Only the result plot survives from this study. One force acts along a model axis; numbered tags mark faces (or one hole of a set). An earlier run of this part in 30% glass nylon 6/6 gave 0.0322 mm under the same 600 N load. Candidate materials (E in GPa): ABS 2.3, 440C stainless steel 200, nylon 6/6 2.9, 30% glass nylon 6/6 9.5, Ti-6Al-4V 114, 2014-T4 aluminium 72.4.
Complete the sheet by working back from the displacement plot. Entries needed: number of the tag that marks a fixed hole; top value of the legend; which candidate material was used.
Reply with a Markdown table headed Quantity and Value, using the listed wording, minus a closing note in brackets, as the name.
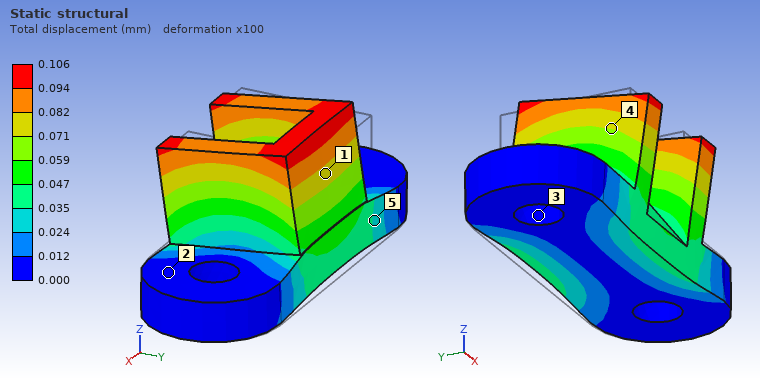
| Quantity | Value |
|---|---|
| number of the tag that marks a fixed hole | 3 |
| top value of the legend | 0.106 mm |
| which candidate material was used | nylon 6/6 |
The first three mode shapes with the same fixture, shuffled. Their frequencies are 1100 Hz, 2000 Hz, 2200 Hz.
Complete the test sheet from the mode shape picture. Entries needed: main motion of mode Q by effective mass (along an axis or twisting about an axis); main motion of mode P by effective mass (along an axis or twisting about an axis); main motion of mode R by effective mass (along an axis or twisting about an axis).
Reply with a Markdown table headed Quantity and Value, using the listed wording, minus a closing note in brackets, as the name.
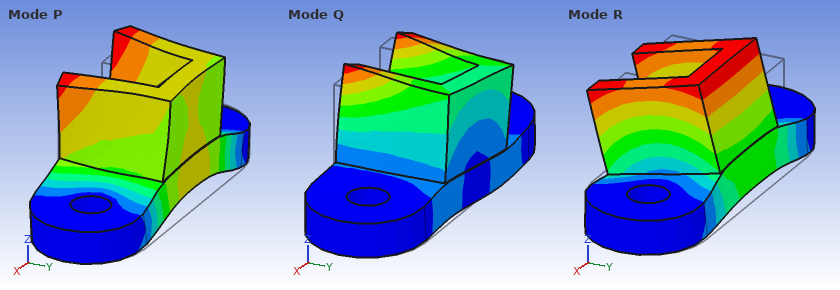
| Quantity | Value |
|---|---|
| main motion of mode Q by effective mass | along X |
| main motion of mode P by effective mass | along Z |
| main motion of mode R by effective mass | along Y |
